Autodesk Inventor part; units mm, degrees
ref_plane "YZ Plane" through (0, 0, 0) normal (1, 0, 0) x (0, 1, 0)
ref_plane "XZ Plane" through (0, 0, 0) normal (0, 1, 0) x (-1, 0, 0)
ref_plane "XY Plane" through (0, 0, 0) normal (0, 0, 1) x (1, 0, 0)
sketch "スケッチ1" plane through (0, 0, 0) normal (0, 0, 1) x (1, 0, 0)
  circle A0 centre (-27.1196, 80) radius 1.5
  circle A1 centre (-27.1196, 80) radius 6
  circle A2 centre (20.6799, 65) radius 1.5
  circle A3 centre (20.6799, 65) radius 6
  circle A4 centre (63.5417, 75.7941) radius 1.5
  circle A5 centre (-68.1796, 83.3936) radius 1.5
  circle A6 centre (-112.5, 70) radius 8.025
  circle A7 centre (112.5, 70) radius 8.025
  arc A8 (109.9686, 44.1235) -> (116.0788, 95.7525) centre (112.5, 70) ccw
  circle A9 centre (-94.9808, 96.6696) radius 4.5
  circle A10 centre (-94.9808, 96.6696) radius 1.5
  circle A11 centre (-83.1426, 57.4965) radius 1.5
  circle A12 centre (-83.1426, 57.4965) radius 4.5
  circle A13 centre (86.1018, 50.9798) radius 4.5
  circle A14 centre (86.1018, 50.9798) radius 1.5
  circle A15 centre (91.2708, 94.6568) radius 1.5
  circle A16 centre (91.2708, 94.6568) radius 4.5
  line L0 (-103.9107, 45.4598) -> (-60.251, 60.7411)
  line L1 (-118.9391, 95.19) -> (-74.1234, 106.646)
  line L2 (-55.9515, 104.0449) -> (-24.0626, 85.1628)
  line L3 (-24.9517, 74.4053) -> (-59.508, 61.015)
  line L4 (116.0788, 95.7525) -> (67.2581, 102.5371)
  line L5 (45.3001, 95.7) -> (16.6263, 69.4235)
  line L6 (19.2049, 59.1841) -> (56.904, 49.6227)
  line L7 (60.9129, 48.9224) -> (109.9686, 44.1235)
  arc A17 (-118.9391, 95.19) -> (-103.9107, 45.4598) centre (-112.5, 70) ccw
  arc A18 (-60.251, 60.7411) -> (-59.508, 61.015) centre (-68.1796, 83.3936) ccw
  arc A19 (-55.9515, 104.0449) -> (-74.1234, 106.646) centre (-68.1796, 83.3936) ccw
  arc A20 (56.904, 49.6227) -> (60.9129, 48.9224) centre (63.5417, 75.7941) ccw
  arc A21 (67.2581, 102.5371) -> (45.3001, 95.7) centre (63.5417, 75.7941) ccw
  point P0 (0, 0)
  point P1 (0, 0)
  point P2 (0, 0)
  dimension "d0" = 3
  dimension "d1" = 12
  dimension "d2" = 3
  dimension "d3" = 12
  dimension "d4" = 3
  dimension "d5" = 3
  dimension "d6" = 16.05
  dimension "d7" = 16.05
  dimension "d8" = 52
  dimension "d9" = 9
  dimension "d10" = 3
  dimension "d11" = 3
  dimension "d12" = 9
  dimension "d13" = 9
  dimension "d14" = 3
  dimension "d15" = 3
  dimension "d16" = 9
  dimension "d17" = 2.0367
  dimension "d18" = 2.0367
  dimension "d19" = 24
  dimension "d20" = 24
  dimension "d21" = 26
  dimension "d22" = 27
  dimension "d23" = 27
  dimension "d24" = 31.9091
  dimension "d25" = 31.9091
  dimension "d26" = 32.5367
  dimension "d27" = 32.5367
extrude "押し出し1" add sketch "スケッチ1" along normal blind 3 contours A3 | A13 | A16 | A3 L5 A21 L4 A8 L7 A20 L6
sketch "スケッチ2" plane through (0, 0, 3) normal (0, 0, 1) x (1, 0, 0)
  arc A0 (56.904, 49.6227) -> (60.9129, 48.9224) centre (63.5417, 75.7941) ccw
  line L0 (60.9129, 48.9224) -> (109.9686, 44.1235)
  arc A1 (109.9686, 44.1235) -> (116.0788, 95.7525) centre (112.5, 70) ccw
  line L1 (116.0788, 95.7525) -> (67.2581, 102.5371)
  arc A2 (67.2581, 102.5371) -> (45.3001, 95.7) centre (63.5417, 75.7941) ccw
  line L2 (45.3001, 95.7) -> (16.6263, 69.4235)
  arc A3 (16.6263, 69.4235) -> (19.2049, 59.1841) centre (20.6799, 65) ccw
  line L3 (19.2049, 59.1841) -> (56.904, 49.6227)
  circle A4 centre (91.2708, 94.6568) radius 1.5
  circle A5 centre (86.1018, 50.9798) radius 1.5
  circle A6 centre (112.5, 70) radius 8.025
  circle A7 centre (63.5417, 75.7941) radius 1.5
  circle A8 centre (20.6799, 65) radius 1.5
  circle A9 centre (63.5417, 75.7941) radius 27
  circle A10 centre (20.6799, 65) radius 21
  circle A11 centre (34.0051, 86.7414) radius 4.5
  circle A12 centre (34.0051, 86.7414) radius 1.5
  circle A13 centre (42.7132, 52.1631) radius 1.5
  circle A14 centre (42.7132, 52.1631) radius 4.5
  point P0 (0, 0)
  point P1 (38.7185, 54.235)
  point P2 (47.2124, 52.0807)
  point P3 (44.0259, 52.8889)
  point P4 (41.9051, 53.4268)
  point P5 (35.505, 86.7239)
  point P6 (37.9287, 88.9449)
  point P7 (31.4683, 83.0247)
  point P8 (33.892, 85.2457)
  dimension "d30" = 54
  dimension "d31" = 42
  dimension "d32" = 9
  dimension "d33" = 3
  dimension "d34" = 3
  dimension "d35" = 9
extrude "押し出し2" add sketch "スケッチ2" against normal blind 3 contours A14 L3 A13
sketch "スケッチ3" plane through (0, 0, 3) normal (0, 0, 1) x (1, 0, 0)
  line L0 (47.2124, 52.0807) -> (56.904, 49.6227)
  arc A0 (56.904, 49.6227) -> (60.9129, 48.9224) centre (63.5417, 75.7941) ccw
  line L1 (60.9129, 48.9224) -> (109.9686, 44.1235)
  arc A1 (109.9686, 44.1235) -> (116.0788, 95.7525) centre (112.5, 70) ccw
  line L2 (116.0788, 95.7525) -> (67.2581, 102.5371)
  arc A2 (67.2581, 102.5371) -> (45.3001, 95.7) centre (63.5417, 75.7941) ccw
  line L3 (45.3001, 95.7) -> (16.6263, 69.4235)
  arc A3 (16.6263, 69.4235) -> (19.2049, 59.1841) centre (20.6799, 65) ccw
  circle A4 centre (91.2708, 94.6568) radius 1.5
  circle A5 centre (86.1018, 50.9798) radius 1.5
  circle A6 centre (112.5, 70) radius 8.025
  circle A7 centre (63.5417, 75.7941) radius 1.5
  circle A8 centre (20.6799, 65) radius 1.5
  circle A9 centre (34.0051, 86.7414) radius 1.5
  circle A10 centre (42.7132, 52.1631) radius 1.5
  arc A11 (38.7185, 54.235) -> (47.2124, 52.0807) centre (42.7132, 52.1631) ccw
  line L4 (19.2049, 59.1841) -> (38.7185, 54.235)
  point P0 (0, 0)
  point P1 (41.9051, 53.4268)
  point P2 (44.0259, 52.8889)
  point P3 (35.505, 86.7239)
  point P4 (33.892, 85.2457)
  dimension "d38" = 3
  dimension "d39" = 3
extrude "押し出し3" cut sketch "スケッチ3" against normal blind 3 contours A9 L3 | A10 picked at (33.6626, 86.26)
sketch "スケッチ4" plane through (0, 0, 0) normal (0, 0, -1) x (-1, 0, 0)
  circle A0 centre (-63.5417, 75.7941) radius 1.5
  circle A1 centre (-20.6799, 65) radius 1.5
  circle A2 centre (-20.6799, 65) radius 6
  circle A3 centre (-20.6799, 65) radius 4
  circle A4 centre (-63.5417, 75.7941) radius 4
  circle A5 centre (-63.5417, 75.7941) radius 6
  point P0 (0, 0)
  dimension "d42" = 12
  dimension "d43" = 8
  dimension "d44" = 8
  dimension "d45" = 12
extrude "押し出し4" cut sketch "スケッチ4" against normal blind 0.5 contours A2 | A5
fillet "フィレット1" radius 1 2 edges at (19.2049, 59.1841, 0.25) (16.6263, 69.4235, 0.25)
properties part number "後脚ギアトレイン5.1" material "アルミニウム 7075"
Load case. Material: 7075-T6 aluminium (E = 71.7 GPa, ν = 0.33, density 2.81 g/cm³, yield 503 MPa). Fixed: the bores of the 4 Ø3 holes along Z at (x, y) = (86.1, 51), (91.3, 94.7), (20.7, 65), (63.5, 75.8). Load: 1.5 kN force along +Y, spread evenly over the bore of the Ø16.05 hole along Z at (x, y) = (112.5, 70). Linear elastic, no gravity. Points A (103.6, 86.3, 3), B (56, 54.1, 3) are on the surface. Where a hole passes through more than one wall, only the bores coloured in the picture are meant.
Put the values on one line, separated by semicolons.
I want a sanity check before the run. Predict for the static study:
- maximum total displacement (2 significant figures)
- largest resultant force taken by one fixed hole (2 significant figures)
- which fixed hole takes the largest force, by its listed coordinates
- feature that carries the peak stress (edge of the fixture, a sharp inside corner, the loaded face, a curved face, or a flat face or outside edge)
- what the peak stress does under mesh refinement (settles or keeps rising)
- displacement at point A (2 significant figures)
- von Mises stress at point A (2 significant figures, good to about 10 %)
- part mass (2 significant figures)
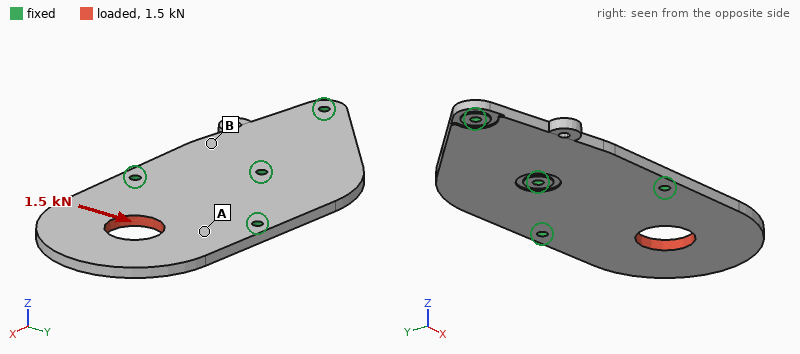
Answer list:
24 µm; 1.1 kN; (91.3, 94.7); edge of the fixture; keeps rising; 8.2 µm; 19 MPa; 43 g
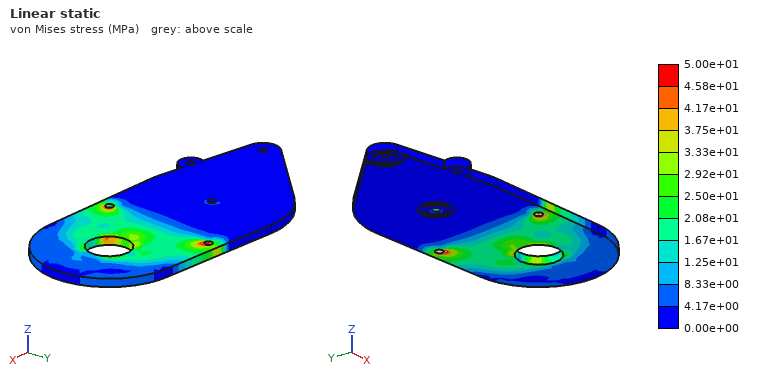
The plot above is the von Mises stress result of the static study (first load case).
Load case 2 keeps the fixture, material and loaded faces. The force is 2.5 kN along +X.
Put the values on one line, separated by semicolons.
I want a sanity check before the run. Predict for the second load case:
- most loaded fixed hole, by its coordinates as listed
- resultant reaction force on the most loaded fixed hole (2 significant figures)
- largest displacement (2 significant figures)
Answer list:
(86.1, 51); 1.2 kN; 14 µm
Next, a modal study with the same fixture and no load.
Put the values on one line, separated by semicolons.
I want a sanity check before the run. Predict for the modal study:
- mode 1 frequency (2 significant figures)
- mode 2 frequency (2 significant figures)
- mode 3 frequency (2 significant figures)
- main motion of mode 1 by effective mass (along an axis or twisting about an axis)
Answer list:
1100 Hz; 3000 Hz; 3800 Hz; along Z
